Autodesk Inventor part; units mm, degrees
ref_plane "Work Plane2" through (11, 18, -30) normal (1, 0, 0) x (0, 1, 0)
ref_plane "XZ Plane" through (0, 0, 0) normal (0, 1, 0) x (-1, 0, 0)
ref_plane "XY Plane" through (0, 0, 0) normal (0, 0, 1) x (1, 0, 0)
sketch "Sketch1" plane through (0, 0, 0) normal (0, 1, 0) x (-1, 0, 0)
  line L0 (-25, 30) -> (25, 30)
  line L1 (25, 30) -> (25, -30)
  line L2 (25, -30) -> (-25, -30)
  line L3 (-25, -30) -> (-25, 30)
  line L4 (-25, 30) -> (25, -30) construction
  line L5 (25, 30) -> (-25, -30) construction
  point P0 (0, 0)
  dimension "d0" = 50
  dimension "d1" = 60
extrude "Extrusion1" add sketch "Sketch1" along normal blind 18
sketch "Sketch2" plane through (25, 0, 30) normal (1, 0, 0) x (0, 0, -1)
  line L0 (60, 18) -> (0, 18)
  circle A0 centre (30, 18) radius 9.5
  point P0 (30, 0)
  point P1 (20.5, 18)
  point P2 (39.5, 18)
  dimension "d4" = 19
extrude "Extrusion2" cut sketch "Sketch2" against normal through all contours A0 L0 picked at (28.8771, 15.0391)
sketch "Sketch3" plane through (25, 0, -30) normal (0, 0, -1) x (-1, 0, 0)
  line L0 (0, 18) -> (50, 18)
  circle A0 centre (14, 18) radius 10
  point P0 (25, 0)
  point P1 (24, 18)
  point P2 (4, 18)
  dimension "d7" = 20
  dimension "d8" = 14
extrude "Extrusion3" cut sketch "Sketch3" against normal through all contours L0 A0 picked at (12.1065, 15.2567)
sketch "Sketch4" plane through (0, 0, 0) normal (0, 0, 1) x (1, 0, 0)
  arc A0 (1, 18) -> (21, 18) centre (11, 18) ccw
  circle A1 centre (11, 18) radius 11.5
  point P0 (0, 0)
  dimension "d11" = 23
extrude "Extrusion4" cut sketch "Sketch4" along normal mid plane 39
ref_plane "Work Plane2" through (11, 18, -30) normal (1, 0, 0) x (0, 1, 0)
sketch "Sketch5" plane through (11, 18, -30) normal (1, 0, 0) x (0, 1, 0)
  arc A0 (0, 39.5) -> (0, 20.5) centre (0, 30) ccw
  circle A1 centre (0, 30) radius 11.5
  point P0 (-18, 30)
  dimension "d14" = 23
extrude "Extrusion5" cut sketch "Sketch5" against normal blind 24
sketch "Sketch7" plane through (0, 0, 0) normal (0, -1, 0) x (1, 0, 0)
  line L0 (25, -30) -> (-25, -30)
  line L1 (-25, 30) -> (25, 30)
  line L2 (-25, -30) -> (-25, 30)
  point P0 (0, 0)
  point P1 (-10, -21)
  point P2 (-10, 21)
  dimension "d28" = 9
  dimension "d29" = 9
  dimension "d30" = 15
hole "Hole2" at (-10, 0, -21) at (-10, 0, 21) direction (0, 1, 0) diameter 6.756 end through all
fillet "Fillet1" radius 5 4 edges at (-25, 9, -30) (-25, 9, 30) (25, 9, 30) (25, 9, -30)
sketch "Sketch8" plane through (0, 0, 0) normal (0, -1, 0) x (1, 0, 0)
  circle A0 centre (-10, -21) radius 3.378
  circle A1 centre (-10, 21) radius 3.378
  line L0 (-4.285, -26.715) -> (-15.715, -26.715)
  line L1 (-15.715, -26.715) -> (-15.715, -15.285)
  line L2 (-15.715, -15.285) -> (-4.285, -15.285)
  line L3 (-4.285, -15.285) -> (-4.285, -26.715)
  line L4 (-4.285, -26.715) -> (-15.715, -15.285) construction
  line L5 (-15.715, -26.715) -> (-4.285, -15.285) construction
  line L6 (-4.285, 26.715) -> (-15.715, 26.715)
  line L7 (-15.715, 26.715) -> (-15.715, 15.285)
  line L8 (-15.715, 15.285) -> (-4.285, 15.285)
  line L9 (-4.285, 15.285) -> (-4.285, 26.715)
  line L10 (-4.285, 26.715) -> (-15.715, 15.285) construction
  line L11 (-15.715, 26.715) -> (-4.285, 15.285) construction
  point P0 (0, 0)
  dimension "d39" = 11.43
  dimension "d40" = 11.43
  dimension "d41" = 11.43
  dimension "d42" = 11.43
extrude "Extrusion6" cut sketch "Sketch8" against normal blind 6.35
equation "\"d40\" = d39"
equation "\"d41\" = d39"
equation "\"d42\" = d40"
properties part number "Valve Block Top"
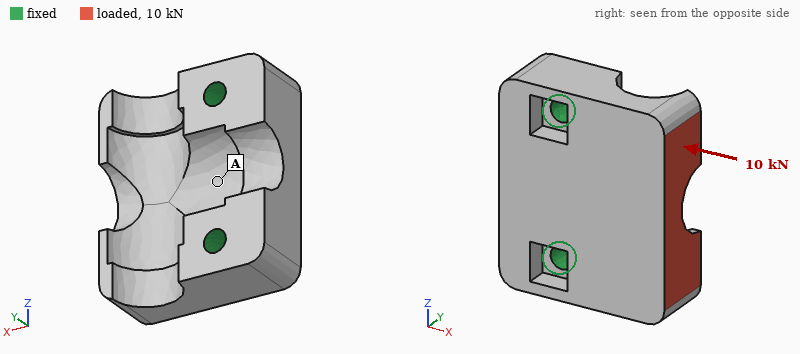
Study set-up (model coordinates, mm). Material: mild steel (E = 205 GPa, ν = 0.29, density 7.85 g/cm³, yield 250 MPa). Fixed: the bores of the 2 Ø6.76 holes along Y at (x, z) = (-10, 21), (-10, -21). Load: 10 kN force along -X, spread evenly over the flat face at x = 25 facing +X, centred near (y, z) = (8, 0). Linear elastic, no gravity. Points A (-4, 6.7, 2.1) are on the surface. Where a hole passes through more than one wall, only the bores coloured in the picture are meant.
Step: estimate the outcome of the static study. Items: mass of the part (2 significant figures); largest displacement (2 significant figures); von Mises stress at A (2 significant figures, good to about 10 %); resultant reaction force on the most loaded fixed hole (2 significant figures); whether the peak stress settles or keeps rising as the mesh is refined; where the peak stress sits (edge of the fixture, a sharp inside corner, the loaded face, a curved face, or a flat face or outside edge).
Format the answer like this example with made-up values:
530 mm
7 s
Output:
270 g
42 µm
20 MPa
5.0 kN
keeps rising
a sharp inside corner
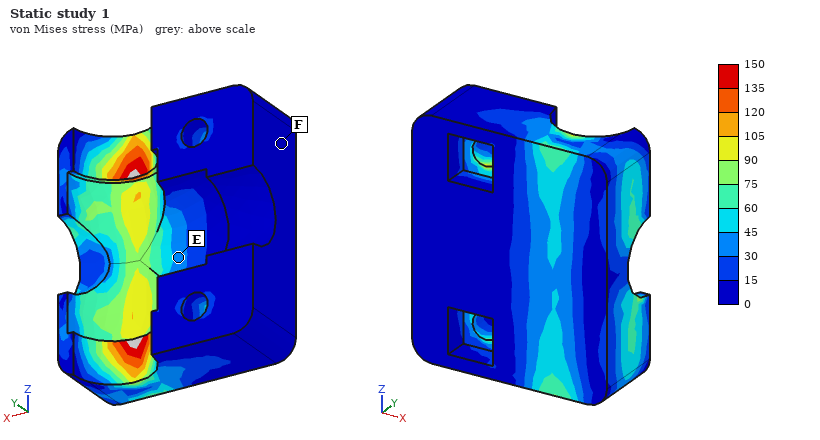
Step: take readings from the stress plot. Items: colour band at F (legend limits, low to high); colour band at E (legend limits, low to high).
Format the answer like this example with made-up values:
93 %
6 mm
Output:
0 to 15 MPa
30 to 45 MPa
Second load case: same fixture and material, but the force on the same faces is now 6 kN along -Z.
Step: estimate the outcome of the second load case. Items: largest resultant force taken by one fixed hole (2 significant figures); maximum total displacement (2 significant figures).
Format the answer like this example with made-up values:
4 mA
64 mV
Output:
5.2 kN
26 µm
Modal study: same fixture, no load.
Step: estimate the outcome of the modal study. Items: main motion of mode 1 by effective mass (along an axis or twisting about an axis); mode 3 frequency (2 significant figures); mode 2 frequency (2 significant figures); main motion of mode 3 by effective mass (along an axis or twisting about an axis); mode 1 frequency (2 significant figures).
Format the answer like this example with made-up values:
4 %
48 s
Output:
along Y
15 kHz
8700 Hz
along Z
5800 Hz
